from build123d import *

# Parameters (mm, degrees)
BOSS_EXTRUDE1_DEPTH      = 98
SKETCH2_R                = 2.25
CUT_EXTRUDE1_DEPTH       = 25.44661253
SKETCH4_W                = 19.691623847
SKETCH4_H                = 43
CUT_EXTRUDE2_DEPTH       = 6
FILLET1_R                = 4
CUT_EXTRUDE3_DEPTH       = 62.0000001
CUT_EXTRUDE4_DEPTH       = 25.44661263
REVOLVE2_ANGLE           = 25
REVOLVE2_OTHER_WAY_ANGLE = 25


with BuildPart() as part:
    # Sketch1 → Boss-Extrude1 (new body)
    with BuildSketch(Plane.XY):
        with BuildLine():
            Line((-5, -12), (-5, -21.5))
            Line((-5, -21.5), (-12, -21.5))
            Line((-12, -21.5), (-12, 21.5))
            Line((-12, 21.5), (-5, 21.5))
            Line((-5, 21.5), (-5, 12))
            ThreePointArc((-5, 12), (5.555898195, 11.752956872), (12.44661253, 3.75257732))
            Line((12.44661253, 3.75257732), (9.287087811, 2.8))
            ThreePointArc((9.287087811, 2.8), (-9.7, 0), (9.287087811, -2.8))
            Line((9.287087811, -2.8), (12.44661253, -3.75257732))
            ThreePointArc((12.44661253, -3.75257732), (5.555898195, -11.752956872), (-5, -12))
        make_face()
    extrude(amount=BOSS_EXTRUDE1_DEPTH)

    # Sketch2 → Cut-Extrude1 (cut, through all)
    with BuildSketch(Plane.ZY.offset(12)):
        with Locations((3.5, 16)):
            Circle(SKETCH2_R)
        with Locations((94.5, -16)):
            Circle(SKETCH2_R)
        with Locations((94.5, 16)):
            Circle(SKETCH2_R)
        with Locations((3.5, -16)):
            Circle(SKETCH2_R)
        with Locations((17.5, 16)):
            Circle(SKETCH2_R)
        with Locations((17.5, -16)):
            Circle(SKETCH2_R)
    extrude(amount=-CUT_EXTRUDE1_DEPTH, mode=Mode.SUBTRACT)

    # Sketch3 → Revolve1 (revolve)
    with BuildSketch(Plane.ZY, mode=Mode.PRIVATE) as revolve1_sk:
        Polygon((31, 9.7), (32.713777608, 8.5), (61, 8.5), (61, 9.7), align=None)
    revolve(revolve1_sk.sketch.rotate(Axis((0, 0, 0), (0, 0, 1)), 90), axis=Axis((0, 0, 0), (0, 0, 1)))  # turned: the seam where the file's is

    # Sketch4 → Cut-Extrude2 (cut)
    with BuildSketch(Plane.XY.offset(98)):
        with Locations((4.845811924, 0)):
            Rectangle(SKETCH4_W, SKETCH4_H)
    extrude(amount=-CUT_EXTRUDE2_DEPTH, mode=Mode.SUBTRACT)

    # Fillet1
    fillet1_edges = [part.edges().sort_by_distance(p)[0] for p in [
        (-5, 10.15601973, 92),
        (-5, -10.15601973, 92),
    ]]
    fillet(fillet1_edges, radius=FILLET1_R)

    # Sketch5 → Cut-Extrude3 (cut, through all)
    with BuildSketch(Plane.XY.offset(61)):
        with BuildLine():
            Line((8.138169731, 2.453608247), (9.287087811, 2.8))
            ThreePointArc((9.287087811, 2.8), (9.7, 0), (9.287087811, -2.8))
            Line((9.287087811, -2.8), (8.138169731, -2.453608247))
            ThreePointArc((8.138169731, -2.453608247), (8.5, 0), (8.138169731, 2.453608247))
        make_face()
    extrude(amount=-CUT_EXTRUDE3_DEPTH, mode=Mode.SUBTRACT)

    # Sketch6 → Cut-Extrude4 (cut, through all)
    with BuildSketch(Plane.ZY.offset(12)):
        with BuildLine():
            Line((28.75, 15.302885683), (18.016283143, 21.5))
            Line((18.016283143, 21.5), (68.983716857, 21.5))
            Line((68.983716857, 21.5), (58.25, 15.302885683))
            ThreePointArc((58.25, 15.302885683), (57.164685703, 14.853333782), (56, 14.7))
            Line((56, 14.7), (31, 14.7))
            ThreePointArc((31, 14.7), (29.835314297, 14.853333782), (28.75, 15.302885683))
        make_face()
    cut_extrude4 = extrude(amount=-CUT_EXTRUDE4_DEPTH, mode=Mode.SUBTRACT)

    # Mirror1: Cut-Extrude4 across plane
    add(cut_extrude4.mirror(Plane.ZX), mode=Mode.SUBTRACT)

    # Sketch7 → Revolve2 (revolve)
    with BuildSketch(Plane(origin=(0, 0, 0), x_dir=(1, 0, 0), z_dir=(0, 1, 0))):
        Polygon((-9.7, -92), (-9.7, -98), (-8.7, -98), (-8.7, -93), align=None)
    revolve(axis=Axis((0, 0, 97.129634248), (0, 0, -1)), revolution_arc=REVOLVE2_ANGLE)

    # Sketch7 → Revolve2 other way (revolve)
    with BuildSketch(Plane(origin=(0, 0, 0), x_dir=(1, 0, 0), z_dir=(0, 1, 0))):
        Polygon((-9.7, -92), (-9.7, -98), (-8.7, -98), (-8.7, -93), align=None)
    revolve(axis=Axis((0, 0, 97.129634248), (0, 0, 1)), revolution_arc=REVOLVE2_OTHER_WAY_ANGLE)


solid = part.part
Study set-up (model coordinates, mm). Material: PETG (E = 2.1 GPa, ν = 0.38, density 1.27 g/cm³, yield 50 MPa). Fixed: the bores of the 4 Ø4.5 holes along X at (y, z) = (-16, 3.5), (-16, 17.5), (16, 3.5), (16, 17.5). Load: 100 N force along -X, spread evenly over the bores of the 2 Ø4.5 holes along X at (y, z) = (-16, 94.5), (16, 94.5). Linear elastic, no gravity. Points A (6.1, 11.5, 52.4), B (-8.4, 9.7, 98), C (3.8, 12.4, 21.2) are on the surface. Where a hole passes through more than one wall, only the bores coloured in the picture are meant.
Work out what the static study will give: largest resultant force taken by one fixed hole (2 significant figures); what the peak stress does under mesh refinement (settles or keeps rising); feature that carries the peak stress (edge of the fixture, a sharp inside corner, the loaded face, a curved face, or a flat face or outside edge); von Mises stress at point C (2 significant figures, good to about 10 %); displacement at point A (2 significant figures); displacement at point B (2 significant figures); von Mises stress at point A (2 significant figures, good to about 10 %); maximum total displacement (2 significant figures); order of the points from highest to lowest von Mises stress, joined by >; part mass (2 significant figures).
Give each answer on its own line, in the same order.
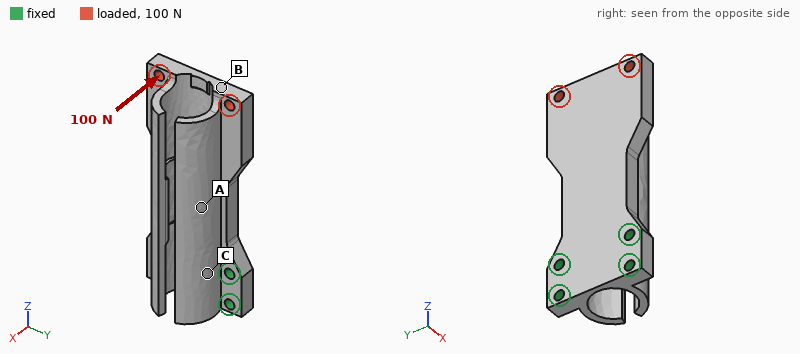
240 N
keeps rising
edge of the fixture
4.8 MPa
0.44 mm
1.1 mm
2.4 MPa
1.2 mm
C > A > B
43 g
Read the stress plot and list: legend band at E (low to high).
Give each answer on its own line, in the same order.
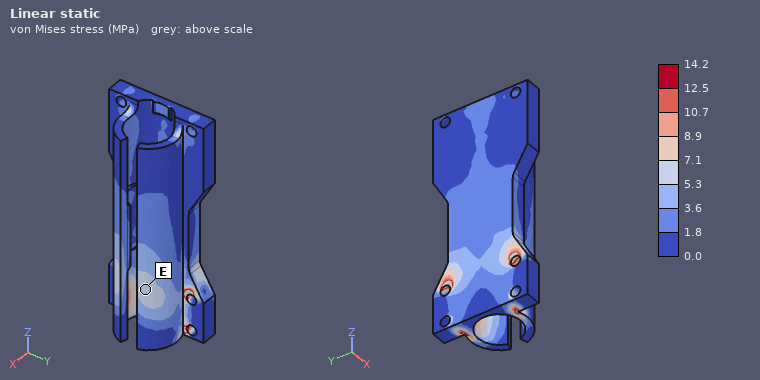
5.3 to 7.1 MPa
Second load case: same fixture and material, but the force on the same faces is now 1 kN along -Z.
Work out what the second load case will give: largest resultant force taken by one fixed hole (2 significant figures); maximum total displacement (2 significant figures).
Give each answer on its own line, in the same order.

400 N
0.52 mm
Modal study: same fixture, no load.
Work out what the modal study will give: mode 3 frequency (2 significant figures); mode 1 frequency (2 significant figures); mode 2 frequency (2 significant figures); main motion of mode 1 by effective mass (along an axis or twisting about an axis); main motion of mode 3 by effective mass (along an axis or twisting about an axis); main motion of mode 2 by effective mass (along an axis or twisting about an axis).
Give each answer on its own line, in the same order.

900 Hz
450 Hz
570 Hz
along X
along Y
along Y
